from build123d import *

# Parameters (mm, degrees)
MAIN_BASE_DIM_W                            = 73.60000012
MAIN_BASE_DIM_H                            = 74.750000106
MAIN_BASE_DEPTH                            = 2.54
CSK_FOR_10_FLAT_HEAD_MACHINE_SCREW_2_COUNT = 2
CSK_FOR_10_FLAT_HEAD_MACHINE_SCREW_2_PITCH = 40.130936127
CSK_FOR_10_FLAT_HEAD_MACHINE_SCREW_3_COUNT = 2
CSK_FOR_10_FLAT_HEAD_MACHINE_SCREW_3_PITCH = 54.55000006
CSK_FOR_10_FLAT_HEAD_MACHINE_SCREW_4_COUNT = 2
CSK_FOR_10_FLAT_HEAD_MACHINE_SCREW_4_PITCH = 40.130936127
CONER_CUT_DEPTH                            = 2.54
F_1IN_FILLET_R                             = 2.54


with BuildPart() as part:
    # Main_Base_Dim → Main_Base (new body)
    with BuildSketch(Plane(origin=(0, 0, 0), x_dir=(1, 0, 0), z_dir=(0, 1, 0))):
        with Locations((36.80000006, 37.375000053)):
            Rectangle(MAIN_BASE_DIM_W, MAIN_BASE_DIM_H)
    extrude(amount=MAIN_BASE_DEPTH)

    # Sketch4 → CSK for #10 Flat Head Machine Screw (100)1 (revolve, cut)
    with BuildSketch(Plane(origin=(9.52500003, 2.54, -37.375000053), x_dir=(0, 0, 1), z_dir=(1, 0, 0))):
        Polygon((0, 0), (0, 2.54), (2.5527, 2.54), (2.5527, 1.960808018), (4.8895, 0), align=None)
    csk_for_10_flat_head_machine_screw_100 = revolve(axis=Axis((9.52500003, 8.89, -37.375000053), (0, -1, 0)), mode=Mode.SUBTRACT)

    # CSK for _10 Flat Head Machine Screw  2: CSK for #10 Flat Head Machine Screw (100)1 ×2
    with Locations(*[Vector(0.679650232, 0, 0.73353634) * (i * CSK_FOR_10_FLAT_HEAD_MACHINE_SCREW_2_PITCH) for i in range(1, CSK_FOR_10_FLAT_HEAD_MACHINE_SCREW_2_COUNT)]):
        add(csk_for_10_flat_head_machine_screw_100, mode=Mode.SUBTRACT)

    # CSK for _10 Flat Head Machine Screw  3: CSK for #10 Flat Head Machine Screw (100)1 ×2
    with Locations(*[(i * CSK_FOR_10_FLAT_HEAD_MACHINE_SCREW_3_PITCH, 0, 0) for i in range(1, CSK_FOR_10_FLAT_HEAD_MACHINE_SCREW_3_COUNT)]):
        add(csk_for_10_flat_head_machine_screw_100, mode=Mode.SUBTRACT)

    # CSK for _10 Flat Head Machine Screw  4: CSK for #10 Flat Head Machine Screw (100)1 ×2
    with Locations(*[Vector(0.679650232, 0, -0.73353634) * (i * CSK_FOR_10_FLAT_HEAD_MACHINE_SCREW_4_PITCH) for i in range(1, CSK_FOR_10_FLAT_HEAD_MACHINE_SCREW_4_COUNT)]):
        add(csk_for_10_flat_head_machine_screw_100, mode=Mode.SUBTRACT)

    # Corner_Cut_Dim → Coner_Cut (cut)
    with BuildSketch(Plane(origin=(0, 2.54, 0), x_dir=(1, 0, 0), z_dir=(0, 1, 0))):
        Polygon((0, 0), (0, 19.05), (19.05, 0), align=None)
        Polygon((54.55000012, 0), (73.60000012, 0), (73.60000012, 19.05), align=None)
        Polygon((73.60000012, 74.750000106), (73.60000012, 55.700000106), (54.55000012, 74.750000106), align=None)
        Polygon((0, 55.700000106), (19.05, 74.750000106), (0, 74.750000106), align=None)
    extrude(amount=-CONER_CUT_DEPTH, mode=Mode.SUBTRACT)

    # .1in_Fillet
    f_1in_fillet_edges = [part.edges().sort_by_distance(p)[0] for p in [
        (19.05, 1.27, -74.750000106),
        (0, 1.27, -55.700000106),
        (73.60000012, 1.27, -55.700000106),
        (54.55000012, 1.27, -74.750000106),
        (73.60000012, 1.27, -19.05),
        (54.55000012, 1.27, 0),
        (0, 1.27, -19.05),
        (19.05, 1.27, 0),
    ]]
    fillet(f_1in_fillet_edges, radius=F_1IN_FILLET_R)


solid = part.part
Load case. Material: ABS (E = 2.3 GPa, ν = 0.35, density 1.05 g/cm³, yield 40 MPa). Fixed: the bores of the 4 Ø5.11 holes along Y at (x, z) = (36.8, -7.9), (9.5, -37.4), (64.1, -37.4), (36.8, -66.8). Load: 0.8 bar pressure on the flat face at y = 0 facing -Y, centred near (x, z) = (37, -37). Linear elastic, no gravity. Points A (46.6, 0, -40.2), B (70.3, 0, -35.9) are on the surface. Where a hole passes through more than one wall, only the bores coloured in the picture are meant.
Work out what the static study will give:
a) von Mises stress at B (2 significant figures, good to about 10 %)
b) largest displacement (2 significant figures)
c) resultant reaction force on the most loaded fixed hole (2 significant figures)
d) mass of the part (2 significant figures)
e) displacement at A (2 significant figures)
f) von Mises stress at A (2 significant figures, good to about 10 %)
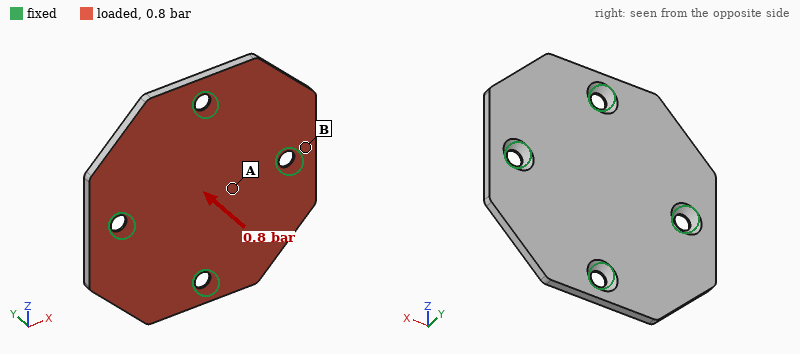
11 MPa
0.65 mm
120 N
12 g
0.30 mm
3.4 MPa
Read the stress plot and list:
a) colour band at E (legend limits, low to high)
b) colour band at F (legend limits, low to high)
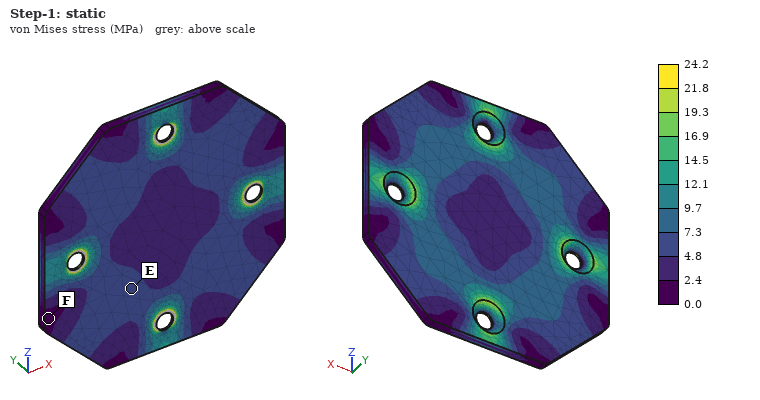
4.8 to 7.3 MPa
0.0 to 2.4 MPa
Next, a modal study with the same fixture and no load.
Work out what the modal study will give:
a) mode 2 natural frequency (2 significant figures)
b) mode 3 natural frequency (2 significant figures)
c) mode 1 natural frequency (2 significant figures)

1200 Hz
1200 Hz
1100 Hz
